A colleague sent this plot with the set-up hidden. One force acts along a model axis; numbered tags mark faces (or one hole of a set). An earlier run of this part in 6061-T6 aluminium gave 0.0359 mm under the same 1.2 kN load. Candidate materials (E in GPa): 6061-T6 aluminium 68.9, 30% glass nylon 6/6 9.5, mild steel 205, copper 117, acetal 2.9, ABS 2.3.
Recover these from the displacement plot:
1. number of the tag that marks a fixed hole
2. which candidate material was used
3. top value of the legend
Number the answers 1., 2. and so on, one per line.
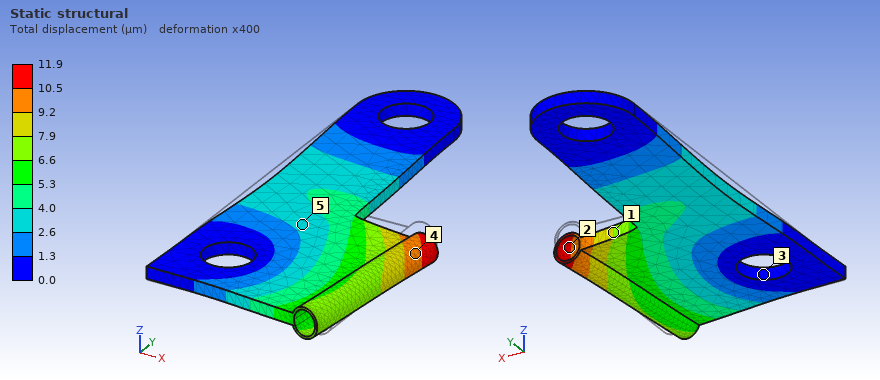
1. 3
2. mild steel
3. 11.9 µm
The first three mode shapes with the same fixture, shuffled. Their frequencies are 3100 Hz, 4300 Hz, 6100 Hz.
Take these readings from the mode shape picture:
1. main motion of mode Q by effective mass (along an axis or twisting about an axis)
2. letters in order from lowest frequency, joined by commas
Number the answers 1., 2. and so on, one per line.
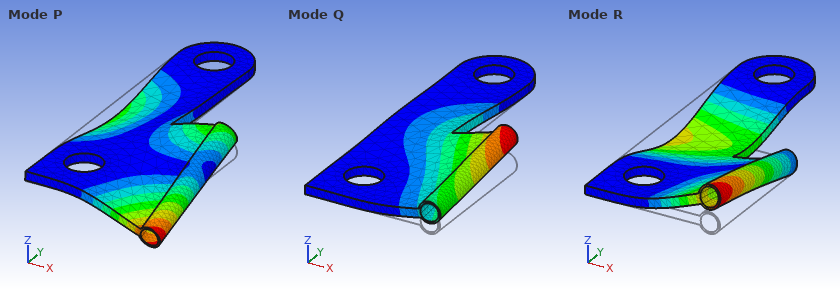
1. along Z
2. Q, R, P
